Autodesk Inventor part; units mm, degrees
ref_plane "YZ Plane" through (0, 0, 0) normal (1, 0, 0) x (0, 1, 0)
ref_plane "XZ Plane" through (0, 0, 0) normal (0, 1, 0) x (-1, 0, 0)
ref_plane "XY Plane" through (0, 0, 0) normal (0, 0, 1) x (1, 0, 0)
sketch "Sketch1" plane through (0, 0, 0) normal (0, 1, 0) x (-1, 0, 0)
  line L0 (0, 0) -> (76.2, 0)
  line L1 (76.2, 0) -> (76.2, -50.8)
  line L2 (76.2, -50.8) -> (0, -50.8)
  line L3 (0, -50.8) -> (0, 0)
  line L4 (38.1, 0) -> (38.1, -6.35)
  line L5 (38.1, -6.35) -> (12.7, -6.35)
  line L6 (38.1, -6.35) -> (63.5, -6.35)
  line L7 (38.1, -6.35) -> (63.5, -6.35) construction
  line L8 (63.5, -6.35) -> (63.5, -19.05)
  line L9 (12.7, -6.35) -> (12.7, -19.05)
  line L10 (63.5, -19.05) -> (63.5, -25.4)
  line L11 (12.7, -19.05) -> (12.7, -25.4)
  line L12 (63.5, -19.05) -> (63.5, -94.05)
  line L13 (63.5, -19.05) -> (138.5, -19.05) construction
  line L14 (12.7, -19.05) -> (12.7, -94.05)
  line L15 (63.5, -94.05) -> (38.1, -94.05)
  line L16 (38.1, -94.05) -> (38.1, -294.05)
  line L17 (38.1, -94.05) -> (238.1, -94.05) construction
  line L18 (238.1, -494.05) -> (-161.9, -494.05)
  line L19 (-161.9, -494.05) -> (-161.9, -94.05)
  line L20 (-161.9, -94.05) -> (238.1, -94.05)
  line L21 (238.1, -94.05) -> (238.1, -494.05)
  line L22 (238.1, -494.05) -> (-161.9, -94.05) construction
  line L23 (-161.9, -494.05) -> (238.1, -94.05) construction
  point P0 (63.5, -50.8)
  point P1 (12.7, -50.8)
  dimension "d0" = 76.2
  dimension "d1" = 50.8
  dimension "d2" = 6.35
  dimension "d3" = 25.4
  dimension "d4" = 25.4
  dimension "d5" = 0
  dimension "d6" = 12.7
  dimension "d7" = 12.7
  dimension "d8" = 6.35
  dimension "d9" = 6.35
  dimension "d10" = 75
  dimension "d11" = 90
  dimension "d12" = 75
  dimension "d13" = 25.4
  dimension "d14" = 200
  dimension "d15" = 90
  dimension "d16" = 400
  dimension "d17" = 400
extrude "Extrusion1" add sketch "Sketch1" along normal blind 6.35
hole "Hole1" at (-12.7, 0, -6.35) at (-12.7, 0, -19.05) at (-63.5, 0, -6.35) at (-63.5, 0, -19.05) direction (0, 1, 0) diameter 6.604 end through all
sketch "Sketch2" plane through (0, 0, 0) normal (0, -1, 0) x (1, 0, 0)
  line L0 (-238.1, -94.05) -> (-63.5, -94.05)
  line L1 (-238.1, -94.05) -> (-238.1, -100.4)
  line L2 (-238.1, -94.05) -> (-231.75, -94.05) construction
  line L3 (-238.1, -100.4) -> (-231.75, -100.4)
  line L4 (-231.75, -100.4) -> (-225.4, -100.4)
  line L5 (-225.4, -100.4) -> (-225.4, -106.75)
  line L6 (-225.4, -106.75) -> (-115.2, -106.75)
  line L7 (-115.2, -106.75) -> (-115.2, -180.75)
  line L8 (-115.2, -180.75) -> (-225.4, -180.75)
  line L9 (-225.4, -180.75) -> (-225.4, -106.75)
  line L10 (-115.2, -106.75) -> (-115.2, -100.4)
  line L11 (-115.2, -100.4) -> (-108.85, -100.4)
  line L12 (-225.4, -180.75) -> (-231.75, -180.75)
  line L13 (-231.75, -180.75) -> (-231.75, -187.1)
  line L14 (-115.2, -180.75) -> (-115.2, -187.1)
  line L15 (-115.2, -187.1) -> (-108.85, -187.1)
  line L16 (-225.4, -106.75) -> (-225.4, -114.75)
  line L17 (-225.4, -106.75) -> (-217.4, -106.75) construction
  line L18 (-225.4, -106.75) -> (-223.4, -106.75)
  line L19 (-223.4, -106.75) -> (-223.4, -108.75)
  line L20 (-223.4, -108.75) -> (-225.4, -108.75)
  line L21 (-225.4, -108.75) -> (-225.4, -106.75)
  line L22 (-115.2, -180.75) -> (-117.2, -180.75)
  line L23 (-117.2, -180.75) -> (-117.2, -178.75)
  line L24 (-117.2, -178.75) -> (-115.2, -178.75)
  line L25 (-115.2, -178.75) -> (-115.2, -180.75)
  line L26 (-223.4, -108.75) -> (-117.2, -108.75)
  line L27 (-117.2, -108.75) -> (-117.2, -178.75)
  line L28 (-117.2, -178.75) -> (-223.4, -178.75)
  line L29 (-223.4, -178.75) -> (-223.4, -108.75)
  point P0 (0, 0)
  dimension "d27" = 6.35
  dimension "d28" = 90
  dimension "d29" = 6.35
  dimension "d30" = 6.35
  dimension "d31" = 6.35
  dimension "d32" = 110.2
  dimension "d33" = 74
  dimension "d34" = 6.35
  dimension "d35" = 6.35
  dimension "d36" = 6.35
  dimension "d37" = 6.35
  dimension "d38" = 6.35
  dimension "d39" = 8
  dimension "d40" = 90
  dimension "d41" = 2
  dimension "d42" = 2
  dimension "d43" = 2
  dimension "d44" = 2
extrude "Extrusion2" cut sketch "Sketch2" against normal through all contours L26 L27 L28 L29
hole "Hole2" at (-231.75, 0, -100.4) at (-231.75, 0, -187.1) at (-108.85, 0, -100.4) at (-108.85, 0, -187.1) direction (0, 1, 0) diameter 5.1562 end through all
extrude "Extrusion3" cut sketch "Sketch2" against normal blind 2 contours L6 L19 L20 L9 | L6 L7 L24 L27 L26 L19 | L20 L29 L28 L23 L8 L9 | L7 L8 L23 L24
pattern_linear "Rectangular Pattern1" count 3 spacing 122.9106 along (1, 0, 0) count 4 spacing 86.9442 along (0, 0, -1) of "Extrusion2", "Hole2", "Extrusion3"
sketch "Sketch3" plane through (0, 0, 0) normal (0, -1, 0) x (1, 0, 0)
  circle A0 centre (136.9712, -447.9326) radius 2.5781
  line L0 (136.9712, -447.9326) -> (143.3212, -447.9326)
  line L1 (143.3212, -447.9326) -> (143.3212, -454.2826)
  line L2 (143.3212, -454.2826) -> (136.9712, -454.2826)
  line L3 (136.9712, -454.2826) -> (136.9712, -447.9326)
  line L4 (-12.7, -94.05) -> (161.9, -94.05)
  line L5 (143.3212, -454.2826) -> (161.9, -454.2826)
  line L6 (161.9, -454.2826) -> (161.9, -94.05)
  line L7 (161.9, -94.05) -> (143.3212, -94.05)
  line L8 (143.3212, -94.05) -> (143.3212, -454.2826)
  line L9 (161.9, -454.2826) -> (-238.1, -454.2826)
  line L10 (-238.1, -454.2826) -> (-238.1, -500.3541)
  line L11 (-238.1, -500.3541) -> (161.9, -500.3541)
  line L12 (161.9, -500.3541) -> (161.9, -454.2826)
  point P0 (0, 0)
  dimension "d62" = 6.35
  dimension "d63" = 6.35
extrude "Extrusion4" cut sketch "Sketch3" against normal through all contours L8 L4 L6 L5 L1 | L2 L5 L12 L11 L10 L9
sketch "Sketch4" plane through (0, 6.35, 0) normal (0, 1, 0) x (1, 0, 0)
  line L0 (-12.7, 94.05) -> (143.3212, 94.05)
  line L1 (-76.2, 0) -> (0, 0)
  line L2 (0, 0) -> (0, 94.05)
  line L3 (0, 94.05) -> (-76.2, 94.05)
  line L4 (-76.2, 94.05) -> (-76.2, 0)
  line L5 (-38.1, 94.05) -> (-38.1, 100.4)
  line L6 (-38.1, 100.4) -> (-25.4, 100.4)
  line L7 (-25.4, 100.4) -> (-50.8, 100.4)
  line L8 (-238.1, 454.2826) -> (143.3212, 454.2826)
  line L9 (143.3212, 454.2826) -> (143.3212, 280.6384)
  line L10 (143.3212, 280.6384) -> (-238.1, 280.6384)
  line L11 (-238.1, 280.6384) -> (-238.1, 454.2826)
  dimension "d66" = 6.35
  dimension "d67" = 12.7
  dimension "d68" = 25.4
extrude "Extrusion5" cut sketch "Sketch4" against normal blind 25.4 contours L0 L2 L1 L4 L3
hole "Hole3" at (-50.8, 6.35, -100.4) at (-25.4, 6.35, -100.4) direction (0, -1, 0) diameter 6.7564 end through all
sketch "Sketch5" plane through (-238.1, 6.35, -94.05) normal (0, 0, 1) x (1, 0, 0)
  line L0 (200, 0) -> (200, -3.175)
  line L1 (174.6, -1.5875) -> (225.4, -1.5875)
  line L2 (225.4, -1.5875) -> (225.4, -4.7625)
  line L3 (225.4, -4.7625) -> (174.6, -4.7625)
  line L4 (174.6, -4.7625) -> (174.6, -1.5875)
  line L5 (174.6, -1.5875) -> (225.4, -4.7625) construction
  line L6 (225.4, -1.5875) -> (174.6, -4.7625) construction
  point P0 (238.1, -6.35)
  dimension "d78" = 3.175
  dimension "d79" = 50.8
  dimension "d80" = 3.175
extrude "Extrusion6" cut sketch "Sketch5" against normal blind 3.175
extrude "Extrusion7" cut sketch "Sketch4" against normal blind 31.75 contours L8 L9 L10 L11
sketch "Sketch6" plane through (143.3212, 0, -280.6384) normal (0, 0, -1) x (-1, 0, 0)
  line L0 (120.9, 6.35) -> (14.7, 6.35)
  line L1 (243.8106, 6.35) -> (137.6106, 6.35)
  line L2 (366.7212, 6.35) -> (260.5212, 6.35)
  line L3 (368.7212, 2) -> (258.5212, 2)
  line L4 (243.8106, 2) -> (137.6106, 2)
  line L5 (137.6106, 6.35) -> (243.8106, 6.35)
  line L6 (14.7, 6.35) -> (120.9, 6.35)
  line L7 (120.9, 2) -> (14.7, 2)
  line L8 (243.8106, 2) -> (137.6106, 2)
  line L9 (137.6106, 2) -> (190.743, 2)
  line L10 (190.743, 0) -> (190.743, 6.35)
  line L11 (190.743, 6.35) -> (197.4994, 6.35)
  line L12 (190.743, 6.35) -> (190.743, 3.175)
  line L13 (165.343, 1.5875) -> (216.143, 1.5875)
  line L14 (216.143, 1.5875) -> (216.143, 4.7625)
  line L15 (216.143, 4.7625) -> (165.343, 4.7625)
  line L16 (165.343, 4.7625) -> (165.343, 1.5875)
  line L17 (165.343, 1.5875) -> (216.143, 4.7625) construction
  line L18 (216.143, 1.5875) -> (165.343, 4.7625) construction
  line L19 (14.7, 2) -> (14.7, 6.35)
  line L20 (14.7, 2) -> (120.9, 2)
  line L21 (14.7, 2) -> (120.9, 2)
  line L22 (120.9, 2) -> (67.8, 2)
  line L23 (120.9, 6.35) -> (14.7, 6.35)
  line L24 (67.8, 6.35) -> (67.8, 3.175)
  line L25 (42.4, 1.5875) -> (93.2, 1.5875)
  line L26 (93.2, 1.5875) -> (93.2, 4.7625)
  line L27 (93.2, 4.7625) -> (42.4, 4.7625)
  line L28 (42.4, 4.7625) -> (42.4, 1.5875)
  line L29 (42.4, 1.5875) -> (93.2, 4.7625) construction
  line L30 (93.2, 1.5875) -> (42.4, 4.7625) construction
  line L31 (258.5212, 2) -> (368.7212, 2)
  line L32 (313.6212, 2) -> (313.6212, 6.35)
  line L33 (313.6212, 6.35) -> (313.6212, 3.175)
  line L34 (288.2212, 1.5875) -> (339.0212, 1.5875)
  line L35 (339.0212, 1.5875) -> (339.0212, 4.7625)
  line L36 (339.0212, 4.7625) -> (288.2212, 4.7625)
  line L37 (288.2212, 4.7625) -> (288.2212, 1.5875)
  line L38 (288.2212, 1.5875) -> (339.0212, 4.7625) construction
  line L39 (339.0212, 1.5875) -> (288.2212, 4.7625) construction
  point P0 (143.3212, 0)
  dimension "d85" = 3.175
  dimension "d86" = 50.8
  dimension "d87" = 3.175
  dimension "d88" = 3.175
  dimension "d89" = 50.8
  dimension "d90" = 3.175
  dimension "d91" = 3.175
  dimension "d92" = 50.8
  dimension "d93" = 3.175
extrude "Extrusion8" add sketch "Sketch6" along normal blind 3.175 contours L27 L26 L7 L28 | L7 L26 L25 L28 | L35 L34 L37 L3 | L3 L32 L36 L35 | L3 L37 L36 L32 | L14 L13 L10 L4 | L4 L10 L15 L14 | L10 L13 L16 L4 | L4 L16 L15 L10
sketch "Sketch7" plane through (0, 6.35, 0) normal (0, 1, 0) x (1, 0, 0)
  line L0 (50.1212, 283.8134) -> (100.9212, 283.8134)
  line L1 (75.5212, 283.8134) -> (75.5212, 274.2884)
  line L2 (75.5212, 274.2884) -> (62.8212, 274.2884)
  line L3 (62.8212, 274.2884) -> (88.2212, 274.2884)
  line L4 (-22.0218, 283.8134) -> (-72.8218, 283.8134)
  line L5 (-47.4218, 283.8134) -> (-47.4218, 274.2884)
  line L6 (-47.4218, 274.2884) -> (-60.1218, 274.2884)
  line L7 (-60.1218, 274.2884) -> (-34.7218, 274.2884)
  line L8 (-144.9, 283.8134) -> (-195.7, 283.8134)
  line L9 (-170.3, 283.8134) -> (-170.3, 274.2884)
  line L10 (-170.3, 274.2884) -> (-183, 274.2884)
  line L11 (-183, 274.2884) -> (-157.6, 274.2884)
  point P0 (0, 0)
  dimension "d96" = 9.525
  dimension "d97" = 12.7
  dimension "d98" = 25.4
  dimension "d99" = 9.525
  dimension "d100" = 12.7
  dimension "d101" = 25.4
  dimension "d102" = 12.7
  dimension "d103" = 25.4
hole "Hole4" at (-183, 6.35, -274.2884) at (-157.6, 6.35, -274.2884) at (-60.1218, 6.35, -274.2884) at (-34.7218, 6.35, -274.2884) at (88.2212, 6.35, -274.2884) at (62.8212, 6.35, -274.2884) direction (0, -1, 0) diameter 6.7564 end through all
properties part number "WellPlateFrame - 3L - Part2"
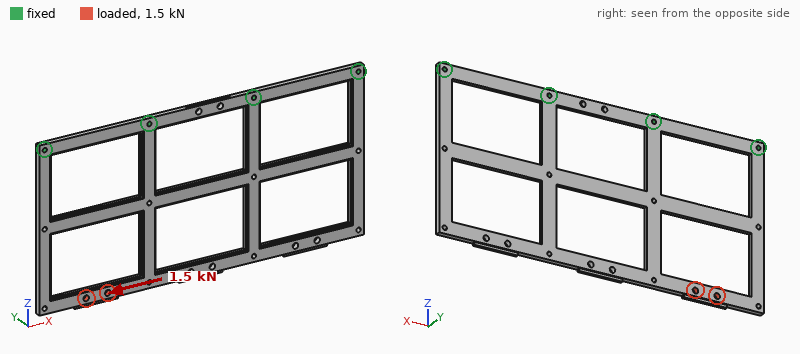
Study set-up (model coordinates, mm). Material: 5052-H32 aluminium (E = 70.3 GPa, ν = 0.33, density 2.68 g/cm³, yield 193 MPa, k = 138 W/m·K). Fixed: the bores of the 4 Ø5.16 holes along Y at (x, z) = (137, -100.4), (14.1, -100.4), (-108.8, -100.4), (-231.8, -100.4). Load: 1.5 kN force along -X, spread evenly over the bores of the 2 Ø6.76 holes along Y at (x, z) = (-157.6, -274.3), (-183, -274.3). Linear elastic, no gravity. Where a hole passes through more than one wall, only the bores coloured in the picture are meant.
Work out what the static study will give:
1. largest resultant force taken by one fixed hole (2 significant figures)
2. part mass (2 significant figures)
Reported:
680 N
420 g
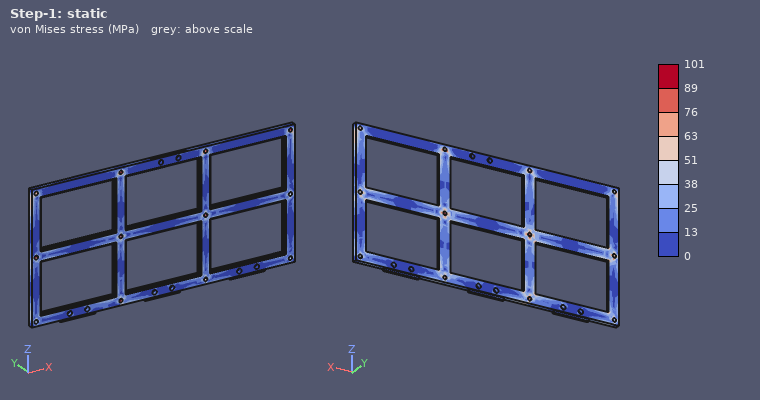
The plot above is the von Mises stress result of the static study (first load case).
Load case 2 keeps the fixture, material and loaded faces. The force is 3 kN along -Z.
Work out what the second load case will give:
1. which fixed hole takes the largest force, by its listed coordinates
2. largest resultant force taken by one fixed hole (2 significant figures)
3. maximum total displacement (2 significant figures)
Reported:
(-108.8, -100.4)
1.6 kN
0.42 mm
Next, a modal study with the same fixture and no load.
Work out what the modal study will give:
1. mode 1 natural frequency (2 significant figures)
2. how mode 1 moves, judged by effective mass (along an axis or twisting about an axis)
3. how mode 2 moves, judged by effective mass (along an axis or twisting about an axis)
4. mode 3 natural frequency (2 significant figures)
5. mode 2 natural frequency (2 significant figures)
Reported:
97 Hz
along Y
twisting about Z
320 Hz
170 Hz
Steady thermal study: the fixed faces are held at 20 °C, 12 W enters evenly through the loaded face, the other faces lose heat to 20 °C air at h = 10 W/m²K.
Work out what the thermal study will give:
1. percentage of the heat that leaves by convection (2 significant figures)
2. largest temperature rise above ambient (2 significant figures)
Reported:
61 %
53 K
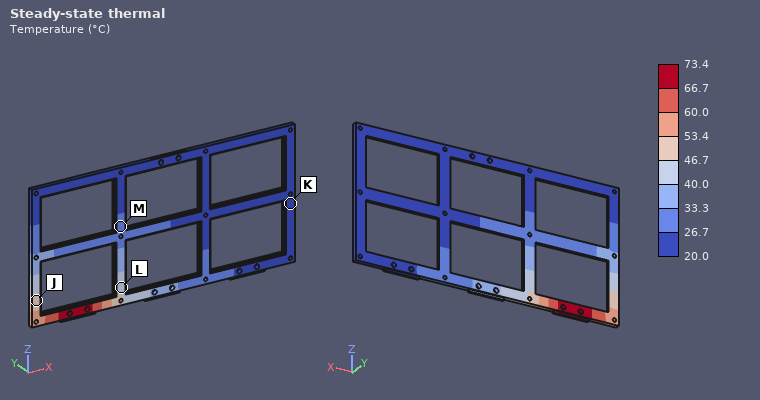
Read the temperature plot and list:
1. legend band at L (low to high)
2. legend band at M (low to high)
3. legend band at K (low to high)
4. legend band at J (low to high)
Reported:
40.0 to 46.7 °C
26.7 to 33.3 °C
20.0 to 26.7 °C
46.7 to 53.4 °C
